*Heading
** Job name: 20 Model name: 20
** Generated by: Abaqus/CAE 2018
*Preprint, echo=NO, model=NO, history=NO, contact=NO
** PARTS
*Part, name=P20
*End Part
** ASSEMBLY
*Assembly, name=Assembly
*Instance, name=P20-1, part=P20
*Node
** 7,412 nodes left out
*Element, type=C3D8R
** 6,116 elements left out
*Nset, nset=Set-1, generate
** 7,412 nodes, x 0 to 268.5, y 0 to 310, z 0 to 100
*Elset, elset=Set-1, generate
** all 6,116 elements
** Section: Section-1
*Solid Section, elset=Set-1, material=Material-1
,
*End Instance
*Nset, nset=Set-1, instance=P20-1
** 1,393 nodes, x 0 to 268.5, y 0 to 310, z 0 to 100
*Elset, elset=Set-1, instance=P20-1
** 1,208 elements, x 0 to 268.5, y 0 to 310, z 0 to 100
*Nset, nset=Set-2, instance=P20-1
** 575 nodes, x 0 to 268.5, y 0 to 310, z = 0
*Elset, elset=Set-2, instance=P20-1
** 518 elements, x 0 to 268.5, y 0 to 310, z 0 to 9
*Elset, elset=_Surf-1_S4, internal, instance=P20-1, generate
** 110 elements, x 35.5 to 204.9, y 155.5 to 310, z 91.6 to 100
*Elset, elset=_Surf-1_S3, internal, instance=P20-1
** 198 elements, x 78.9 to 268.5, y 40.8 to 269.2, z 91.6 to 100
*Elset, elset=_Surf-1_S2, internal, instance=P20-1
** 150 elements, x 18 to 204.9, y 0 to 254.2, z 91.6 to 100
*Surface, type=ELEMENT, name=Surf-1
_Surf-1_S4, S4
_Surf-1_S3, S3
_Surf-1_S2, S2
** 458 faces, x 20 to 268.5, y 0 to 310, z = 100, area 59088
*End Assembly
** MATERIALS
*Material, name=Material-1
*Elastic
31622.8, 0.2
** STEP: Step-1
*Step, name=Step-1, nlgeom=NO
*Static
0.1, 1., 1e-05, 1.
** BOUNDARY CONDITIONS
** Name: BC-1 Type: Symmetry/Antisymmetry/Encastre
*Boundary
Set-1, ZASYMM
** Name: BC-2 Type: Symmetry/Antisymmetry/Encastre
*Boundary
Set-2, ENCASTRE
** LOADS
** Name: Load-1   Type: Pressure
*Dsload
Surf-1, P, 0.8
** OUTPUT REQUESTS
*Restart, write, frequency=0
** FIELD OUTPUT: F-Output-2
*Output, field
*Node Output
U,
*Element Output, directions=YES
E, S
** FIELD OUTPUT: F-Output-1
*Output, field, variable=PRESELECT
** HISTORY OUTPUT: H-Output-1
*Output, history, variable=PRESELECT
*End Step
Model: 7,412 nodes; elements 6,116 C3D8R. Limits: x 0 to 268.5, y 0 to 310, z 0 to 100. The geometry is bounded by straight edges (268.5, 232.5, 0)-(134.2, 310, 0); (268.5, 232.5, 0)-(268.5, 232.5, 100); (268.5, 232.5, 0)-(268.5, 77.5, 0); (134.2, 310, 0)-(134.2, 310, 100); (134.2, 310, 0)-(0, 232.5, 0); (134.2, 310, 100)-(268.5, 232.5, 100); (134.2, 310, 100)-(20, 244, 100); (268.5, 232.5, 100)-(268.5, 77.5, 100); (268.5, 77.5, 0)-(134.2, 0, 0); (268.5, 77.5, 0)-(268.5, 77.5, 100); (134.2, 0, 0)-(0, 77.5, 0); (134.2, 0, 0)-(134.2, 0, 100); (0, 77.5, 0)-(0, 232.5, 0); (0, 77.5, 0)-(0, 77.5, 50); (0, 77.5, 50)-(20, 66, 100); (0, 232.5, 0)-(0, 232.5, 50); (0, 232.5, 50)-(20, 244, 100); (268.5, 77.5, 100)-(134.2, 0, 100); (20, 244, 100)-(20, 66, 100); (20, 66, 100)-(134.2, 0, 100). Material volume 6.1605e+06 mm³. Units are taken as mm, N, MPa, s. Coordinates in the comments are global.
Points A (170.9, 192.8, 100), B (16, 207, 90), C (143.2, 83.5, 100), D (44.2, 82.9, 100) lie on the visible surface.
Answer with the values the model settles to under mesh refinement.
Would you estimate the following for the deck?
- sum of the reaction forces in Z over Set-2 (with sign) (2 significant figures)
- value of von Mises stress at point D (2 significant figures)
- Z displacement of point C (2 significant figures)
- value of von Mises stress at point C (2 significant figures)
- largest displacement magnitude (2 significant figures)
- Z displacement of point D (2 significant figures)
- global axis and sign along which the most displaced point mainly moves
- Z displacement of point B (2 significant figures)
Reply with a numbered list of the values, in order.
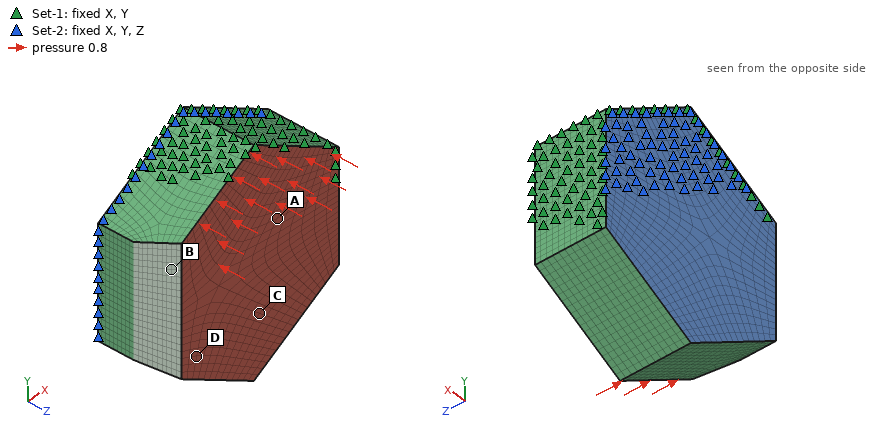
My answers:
1. 47000 N
2. 0.57 MPa
3. -0.0023 mm
4. 0.60 MPa
5. 0.0023 mm
6. -0.0020 mm
7. -Z
8. -0.0013 mm
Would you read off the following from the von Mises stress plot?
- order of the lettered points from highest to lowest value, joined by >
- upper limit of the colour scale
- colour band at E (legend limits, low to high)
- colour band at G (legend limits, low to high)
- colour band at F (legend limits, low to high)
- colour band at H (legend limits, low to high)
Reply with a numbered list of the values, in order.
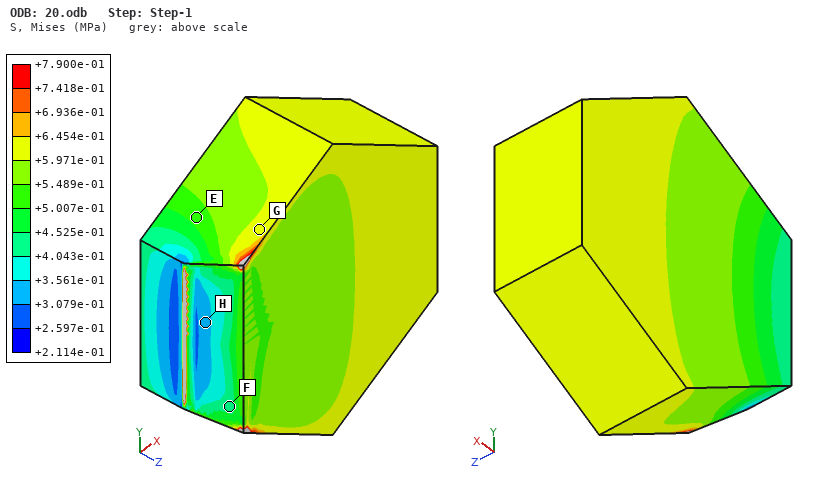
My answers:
1. G > E > F > H
2. +7.900e-01 MPa
3. +5.007e-01 to +5.489e-01 MPa
4. +5.971e-01 to +6.454e-01 MPa
5. +4.043e-01 to +4.525e-01 MPa
6. +3.079e-01 to +3.561e-01 MPa
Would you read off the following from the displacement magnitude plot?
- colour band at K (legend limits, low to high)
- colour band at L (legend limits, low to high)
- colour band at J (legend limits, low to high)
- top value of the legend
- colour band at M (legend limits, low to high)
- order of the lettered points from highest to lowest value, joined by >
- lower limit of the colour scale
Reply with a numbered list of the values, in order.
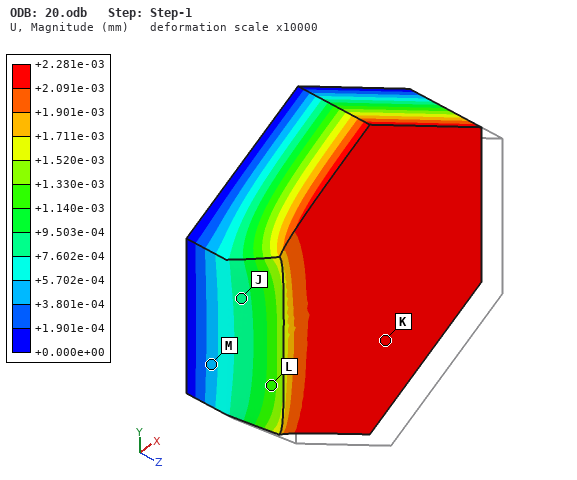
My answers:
1. +2.091e-03 to +2.281e-03 mm
2. +1.140e-03 to +1.330e-03 mm
3. +7.602e-04 to +9.503e-04 mm
4. +2.281e-03 mm
5. +3.801e-04 to +5.702e-04 mm
6. K > L > J > M
7. +0.000e+00 mm
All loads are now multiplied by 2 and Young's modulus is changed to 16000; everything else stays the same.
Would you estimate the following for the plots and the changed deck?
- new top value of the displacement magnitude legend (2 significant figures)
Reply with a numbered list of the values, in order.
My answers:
1. 0.0090 mm
